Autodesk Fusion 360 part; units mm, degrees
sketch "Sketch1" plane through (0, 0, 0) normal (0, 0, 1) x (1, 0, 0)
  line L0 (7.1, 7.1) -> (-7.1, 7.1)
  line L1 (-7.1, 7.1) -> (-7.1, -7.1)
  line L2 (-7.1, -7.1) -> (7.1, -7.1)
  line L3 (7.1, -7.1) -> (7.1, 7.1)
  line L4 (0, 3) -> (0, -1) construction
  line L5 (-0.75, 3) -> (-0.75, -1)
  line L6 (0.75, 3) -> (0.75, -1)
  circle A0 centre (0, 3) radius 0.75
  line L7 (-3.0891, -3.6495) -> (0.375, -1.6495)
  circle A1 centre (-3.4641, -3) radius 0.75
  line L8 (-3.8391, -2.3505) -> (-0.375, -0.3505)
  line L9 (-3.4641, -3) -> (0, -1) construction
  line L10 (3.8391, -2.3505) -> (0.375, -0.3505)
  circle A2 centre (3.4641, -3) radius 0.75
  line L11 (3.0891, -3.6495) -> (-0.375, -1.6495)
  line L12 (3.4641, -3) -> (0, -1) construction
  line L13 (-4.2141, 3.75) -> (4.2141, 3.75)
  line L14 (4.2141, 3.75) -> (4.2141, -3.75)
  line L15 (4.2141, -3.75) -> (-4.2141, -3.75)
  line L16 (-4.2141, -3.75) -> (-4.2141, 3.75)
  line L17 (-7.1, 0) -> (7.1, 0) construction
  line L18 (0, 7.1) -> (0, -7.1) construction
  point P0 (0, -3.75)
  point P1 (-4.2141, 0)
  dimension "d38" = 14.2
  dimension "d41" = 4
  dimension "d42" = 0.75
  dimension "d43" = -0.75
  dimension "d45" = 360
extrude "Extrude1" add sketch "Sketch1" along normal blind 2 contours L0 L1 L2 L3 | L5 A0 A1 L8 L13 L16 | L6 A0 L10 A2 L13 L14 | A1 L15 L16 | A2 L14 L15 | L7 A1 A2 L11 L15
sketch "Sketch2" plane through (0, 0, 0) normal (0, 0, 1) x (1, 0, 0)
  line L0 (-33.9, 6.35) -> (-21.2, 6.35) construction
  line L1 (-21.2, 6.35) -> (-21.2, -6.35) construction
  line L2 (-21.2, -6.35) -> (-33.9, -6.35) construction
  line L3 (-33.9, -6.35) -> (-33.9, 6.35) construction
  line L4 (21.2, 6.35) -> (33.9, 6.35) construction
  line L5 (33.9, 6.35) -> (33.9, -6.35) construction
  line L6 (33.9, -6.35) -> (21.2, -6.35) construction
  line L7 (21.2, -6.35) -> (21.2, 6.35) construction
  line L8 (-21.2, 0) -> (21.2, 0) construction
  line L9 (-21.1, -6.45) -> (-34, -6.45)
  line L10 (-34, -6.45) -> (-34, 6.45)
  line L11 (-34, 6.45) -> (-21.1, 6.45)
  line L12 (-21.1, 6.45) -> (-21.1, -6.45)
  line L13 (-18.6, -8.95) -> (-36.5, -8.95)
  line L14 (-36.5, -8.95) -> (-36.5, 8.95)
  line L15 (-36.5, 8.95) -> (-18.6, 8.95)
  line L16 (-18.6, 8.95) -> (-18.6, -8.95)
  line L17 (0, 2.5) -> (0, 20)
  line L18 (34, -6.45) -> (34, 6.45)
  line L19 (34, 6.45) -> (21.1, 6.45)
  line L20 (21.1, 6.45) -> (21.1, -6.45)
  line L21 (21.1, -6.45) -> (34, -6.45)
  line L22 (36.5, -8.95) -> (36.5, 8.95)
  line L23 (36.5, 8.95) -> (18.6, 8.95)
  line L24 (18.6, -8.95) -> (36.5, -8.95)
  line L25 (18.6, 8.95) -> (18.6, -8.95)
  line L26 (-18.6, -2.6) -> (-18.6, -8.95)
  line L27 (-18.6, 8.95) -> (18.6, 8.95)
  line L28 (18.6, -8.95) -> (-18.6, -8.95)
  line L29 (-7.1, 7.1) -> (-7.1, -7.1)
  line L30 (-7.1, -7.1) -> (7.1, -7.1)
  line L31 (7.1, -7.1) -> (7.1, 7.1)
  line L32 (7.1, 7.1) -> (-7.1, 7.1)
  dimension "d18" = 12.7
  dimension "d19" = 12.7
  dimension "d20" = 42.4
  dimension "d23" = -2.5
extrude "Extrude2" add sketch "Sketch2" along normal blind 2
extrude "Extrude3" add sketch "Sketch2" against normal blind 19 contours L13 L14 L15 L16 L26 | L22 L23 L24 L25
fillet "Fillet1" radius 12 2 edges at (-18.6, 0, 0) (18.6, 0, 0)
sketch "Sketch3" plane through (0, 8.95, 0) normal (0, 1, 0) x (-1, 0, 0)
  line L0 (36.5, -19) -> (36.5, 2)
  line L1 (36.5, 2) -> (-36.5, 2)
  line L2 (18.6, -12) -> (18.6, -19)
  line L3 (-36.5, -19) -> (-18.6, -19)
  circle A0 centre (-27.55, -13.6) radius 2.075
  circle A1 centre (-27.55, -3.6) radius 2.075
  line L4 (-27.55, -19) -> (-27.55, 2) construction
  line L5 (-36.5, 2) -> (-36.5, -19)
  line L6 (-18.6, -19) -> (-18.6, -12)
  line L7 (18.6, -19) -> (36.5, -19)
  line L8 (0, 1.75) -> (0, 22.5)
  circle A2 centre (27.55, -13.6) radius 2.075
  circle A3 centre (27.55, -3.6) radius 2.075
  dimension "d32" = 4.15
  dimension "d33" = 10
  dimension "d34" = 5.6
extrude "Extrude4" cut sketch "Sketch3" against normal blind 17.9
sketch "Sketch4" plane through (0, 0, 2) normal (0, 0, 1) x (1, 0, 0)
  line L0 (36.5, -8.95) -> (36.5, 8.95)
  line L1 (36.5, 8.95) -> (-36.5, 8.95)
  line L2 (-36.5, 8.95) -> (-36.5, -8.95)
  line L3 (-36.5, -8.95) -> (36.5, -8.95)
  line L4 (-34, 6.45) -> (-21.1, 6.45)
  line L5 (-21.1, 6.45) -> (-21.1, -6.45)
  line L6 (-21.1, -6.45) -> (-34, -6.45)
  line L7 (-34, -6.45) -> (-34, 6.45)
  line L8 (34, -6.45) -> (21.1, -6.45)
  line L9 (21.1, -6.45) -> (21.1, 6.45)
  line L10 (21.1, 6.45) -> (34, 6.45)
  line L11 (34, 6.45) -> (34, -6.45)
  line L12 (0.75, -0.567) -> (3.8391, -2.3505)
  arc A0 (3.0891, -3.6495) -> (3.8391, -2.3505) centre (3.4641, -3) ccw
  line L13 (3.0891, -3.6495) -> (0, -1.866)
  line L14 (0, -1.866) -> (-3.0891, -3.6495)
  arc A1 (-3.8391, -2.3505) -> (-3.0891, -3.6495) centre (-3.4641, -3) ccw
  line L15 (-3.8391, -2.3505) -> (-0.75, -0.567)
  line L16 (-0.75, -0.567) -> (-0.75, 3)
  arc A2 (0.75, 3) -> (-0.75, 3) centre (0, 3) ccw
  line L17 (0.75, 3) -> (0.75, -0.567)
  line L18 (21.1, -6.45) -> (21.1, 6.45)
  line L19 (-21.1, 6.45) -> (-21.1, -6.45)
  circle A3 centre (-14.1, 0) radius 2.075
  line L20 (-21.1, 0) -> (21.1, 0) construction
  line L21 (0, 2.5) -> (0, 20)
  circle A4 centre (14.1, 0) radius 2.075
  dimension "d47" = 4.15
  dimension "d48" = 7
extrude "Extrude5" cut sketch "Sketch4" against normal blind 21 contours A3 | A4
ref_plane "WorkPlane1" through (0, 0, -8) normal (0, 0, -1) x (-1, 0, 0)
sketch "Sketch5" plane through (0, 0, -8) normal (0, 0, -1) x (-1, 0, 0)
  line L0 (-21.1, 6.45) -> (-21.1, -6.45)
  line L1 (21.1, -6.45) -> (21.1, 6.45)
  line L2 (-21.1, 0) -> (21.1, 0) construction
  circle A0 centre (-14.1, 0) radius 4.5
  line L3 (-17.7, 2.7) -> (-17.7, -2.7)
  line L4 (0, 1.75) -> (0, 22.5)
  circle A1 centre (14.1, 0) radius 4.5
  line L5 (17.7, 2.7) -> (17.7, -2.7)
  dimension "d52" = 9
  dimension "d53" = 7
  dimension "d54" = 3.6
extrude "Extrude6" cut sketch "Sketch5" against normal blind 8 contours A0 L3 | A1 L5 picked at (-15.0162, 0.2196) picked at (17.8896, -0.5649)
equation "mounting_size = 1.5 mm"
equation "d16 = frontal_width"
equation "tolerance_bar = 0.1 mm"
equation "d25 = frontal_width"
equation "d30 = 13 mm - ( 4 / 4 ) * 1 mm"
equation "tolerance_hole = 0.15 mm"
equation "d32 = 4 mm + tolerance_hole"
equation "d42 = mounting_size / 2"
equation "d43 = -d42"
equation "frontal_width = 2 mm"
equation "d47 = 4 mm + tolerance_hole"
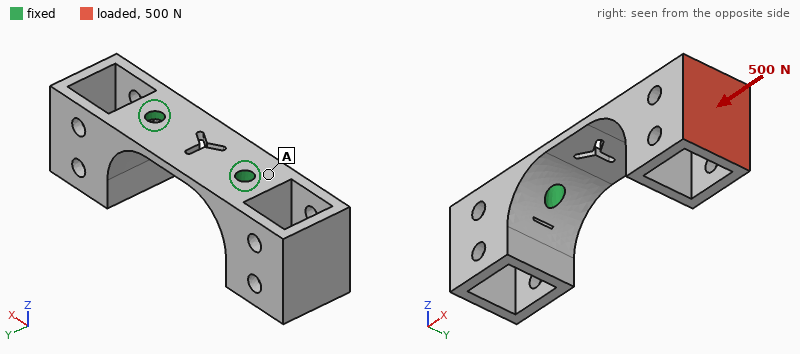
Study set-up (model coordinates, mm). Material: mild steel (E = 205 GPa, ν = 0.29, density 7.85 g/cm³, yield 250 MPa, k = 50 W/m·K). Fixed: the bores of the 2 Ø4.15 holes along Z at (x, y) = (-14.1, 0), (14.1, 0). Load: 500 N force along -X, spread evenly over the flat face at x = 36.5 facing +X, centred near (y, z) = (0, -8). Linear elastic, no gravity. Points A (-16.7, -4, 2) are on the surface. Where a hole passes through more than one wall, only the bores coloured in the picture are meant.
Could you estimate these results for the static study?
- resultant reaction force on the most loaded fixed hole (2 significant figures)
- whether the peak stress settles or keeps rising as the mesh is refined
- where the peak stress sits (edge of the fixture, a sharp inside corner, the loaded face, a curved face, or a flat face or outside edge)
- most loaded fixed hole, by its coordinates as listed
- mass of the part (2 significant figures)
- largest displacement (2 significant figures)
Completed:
400 N
keeps rising
edge of the fixture
(14.1, 0)
65 g
64 µm
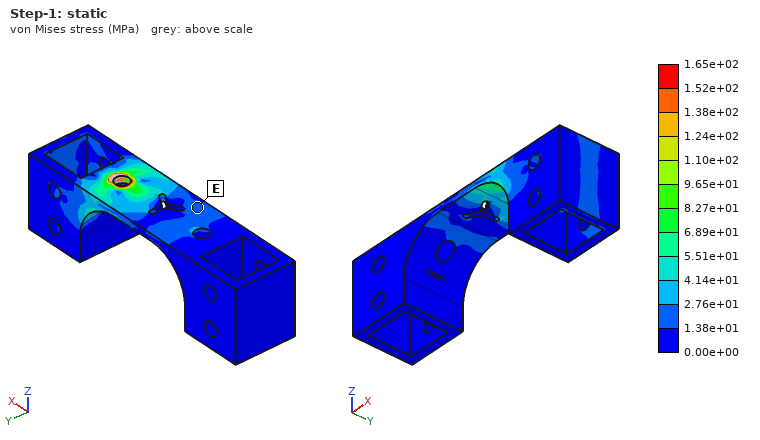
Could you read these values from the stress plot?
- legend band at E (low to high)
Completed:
1.38e+01 to 2.76e+01 MPa
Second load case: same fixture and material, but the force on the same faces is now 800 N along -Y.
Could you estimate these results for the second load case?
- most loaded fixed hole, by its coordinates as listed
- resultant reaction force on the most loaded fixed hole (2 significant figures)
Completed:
(14.1, 0)
1.2 kN
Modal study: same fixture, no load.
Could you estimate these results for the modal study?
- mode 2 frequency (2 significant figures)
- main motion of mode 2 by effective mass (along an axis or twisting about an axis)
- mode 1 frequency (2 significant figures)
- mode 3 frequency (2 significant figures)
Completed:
3800 Hz
along Y
2600 Hz
4800 Hz
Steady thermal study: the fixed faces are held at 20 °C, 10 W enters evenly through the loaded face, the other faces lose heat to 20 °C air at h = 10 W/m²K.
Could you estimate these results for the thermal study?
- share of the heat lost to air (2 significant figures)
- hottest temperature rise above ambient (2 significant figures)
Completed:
12 %
69 K
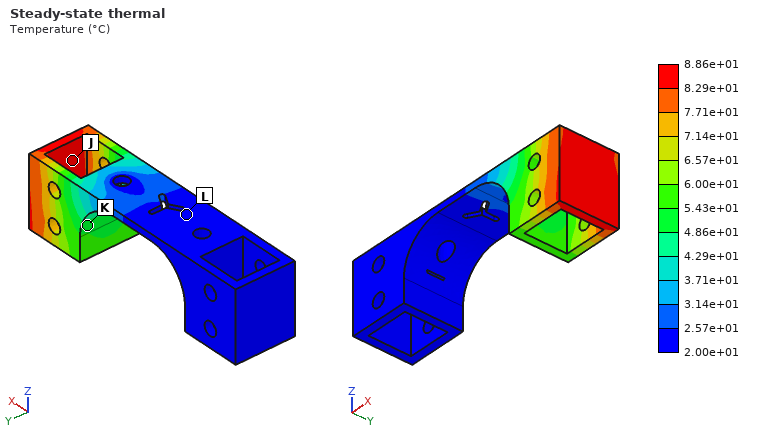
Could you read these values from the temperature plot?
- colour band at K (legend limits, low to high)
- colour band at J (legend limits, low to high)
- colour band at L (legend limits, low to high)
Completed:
4.86e+01 to 5.43e+01 °C
8.29e+01 to 8.86e+01 °C
2.00e+01 to 2.57e+01 °C
